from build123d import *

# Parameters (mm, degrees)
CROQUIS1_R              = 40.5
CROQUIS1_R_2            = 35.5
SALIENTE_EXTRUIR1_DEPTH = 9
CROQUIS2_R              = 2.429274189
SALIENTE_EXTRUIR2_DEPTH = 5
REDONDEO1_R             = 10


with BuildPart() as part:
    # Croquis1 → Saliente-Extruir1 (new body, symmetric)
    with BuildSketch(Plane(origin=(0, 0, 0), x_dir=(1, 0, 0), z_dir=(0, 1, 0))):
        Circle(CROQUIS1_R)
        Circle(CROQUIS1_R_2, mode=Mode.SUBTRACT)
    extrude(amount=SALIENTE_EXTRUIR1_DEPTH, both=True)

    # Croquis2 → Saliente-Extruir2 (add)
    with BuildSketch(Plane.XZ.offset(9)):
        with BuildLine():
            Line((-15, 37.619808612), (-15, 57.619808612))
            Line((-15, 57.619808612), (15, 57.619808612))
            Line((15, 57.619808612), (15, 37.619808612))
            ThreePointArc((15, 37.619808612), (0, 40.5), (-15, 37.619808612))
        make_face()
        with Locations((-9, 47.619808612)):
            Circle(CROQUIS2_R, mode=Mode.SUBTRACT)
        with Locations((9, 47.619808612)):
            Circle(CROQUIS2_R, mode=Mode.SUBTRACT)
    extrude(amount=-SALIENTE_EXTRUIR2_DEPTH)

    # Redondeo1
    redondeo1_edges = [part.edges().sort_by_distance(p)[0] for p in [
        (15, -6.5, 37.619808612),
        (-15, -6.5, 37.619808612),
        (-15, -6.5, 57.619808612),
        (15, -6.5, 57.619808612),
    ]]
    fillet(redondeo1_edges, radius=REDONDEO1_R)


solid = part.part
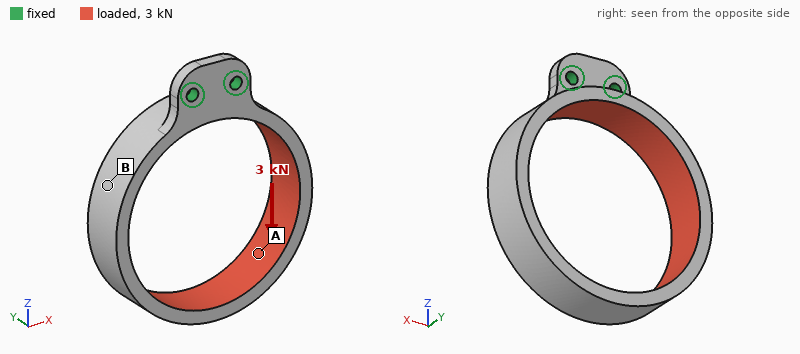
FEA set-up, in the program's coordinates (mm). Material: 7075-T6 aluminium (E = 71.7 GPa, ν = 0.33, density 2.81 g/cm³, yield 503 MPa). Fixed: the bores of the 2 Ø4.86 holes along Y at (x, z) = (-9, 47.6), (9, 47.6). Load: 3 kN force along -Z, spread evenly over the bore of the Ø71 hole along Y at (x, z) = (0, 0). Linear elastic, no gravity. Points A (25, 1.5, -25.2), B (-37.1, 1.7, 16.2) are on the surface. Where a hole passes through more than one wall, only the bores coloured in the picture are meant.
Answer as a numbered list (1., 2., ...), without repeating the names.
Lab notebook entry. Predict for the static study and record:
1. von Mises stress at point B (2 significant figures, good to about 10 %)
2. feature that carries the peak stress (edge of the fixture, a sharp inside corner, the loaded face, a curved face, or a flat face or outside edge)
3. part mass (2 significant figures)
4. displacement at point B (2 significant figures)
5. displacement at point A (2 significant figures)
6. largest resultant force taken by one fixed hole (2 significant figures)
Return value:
1. 77 MPa
2. a sharp inside corner
3. 67 g
4. 0.49 mm
5. 0.89 mm
6. 1.8 kN
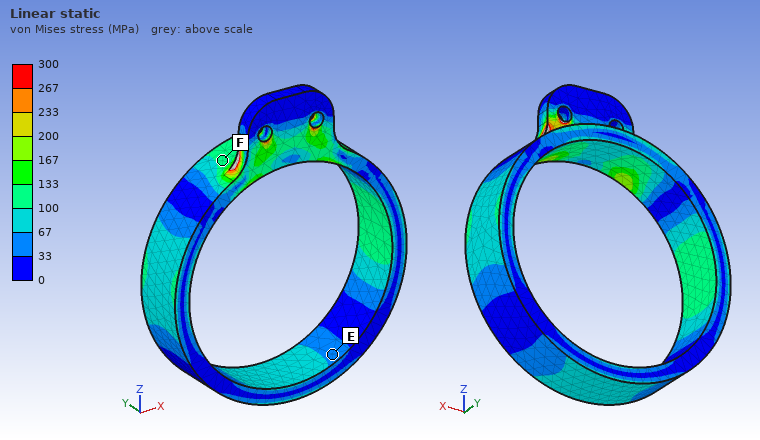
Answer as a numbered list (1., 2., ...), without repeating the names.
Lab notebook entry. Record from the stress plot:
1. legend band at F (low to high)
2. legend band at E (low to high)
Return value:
1. 100 to 133 MPa
2. 33 to 67 MPa
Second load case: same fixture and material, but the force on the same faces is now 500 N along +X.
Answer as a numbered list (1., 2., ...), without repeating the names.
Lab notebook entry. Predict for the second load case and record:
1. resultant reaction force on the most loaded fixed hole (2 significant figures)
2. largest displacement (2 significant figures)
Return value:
1. 1.1 kN
2. 0.70 mm
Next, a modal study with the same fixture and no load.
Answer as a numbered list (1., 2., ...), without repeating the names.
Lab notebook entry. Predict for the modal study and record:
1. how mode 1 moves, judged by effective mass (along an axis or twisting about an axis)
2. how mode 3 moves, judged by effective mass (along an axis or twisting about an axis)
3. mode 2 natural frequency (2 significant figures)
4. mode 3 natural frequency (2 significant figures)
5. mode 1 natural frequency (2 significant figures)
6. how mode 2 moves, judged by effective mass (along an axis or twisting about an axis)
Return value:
1. along Y
2. twisting about Z
3. 590 Hz
4. 1400 Hz
5. 480 Hz
6. along X
